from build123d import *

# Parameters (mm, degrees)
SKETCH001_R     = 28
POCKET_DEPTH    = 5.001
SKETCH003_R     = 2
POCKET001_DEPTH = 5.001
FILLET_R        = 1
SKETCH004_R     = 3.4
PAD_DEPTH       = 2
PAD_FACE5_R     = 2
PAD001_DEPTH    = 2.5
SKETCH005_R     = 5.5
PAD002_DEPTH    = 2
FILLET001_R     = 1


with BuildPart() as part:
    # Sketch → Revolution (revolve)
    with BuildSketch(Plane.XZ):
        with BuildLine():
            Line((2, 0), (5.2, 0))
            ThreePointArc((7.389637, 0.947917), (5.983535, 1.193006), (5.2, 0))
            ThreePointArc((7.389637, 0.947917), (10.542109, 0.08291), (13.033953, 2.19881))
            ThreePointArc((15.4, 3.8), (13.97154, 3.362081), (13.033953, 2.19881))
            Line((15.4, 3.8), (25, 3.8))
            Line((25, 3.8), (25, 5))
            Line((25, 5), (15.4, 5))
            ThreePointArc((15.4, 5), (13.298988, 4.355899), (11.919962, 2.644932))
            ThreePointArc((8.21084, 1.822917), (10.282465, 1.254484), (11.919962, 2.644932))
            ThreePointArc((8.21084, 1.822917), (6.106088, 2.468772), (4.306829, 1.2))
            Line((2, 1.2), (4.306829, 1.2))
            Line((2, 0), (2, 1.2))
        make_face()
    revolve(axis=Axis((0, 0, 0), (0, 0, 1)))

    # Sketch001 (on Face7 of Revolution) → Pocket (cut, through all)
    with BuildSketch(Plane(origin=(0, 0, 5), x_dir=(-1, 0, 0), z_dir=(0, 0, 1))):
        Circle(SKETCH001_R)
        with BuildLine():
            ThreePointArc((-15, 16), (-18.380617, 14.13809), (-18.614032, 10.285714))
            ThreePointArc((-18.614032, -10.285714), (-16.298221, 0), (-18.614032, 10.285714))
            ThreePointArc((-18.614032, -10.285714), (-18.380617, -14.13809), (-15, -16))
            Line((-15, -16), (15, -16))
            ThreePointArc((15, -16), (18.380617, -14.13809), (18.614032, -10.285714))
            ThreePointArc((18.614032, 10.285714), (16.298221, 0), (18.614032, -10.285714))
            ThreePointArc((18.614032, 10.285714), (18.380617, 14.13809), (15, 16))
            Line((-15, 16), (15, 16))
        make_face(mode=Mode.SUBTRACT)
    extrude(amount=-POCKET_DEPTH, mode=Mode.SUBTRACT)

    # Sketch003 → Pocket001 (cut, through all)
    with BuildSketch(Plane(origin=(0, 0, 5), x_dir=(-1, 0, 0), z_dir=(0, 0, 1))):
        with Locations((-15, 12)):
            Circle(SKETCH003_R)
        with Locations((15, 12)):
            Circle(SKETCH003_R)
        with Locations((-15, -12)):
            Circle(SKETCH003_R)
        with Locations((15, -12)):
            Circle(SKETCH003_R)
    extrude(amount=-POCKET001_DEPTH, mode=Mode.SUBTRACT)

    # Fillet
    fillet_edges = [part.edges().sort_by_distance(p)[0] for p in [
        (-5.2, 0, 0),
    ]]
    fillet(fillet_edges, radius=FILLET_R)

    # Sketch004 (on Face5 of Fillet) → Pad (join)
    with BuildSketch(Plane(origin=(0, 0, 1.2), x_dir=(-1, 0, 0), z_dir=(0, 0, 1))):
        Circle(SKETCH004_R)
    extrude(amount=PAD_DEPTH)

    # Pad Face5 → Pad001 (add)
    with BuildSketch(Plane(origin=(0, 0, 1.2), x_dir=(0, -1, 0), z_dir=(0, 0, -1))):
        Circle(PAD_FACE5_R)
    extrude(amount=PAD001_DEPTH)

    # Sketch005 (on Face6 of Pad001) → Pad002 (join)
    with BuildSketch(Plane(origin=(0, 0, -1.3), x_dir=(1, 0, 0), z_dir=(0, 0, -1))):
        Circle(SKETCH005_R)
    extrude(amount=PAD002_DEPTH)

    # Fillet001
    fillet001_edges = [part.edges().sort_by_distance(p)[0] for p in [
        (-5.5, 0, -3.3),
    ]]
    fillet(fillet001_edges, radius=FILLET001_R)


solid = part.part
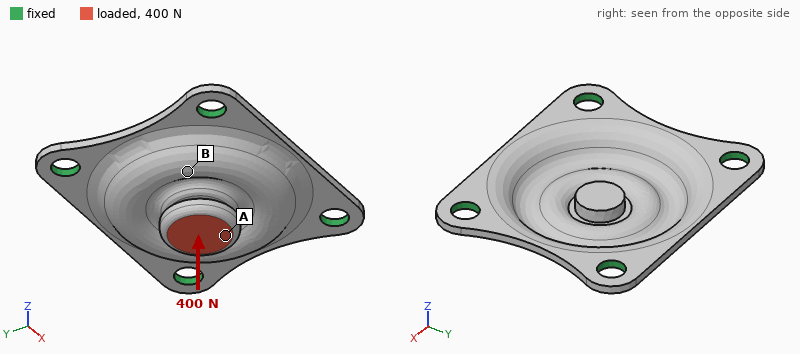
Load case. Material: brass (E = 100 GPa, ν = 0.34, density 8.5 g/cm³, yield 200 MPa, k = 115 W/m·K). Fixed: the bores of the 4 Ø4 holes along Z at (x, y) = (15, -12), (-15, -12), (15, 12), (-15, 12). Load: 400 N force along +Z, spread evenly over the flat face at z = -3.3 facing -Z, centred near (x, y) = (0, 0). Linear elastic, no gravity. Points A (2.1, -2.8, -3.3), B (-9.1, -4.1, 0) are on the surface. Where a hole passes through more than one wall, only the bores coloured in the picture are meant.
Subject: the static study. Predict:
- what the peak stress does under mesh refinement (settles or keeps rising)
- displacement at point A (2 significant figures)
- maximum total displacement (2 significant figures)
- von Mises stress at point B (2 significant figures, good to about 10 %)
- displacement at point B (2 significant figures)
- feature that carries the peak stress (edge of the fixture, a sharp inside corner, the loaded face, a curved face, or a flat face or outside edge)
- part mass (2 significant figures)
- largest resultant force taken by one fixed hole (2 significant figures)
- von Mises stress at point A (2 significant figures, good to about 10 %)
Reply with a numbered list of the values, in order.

1. keeps rising
2. 42 µm
3. 43 µm
4. 63 MPa
5. 14 µm
6. edge of the fixture
7. 15 g
8. 220 N
9. 18 MPa
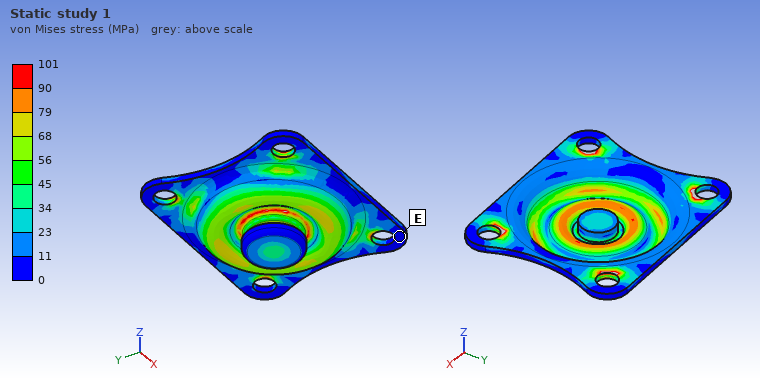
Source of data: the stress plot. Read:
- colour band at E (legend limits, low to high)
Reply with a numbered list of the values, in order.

1. 0 to 11 MPa
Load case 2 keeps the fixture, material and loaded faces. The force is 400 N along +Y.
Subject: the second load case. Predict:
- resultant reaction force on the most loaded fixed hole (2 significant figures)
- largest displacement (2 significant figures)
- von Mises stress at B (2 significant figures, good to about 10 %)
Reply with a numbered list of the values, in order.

1. 160 N
2. 53 µm
3. 30 MPa
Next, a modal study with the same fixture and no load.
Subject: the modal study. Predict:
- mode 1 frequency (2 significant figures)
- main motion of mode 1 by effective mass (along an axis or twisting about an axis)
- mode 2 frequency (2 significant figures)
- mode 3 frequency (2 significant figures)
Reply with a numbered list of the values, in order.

1. 7300 Hz
2. along Z
3. 10000 Hz
4. 12 kHz
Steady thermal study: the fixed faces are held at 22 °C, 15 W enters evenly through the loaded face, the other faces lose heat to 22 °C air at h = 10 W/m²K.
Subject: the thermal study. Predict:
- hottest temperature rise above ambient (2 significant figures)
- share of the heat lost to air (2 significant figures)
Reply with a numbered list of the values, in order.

1. 78 K
2. 3.7 %
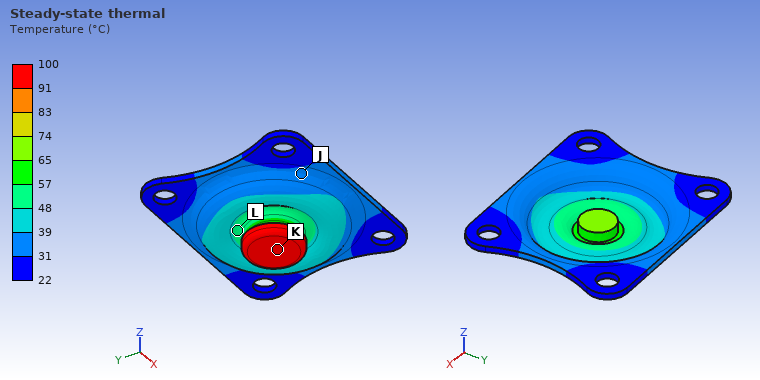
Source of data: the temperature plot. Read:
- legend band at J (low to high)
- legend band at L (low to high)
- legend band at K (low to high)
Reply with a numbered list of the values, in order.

1. 31 to 39 °C
2. 48 to 57 °C
3. 91 to 100 °C
